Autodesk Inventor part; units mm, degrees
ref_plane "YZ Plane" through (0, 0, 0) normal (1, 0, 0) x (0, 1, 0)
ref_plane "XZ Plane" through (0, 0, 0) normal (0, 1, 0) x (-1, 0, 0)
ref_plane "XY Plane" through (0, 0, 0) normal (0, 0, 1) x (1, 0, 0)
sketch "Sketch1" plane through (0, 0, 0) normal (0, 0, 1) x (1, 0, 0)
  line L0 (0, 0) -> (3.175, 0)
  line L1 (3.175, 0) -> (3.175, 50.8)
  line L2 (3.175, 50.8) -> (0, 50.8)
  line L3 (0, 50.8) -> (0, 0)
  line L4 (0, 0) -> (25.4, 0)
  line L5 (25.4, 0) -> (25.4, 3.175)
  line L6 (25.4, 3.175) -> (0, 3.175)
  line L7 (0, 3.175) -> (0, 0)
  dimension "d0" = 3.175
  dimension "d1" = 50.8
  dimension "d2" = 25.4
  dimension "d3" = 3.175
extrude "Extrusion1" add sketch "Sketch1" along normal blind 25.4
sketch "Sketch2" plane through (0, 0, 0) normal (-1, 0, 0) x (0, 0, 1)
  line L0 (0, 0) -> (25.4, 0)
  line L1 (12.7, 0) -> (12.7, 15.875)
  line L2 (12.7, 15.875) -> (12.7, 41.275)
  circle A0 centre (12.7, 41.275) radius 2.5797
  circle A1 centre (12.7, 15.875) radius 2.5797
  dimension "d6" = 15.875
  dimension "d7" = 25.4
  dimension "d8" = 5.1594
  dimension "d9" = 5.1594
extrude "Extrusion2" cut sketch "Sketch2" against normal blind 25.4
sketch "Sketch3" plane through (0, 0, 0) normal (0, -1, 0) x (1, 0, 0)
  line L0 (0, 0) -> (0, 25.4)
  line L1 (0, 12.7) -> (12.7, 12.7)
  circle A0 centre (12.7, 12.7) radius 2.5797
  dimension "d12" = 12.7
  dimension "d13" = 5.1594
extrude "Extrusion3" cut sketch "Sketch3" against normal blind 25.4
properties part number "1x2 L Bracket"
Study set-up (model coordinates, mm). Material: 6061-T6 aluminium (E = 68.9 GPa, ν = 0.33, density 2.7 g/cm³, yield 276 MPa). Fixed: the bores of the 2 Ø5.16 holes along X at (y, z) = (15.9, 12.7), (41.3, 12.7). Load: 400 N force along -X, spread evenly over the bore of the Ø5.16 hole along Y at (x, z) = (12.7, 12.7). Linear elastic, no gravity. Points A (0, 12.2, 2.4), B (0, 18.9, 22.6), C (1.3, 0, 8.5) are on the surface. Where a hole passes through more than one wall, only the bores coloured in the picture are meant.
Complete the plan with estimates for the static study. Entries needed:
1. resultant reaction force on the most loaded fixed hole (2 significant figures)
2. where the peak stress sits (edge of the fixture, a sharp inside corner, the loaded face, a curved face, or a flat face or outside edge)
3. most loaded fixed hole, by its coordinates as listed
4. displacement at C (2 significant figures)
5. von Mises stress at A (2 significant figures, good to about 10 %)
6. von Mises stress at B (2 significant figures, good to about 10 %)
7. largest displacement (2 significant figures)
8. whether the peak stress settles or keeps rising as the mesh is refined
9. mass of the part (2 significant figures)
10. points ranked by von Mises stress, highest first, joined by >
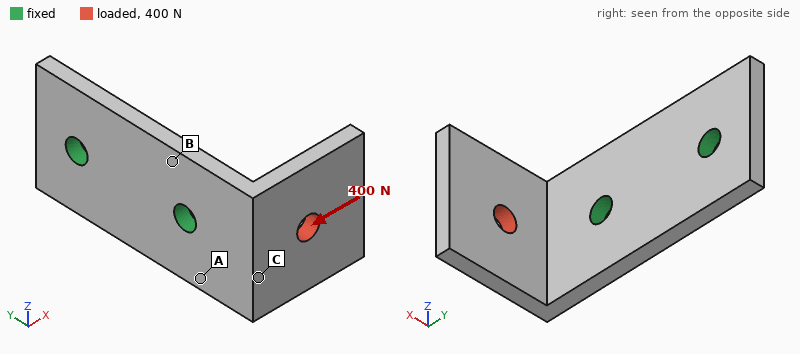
440 N
edge of the fixture
(15.9, 12.7)
0.089 mm
60 MPa
28 MPa
0.21 mm
keeps rising
15 g
A > B > C
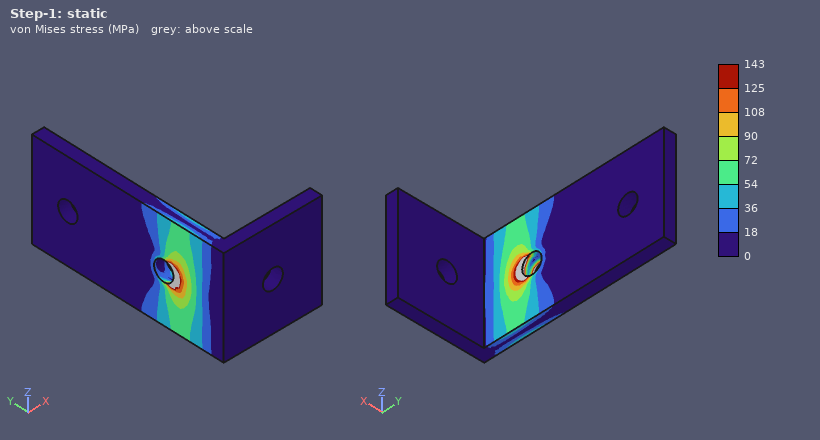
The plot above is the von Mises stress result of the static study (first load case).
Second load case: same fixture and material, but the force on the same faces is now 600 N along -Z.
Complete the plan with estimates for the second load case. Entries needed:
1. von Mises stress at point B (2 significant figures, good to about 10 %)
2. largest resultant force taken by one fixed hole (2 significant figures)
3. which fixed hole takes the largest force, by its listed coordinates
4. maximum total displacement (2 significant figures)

73 MPa
830 N
(15.9, 12.7)
0.29 mm
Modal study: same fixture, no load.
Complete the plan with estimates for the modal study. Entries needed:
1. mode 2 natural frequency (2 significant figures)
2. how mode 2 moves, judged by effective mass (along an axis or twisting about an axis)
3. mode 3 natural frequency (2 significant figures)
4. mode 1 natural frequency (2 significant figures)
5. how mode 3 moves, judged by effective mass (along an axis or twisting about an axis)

3500 Hz
along Z
7200 Hz
2400 Hz
along X
